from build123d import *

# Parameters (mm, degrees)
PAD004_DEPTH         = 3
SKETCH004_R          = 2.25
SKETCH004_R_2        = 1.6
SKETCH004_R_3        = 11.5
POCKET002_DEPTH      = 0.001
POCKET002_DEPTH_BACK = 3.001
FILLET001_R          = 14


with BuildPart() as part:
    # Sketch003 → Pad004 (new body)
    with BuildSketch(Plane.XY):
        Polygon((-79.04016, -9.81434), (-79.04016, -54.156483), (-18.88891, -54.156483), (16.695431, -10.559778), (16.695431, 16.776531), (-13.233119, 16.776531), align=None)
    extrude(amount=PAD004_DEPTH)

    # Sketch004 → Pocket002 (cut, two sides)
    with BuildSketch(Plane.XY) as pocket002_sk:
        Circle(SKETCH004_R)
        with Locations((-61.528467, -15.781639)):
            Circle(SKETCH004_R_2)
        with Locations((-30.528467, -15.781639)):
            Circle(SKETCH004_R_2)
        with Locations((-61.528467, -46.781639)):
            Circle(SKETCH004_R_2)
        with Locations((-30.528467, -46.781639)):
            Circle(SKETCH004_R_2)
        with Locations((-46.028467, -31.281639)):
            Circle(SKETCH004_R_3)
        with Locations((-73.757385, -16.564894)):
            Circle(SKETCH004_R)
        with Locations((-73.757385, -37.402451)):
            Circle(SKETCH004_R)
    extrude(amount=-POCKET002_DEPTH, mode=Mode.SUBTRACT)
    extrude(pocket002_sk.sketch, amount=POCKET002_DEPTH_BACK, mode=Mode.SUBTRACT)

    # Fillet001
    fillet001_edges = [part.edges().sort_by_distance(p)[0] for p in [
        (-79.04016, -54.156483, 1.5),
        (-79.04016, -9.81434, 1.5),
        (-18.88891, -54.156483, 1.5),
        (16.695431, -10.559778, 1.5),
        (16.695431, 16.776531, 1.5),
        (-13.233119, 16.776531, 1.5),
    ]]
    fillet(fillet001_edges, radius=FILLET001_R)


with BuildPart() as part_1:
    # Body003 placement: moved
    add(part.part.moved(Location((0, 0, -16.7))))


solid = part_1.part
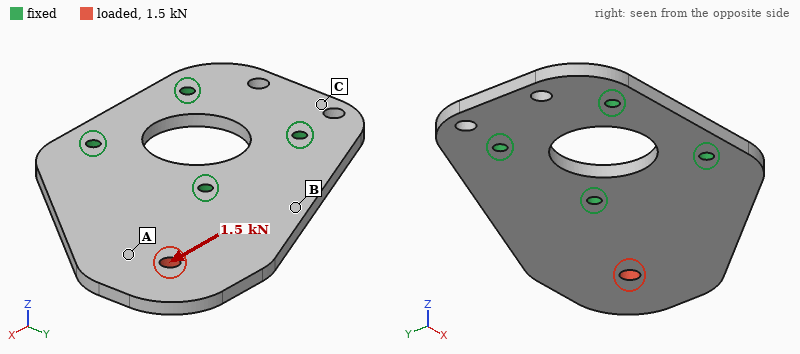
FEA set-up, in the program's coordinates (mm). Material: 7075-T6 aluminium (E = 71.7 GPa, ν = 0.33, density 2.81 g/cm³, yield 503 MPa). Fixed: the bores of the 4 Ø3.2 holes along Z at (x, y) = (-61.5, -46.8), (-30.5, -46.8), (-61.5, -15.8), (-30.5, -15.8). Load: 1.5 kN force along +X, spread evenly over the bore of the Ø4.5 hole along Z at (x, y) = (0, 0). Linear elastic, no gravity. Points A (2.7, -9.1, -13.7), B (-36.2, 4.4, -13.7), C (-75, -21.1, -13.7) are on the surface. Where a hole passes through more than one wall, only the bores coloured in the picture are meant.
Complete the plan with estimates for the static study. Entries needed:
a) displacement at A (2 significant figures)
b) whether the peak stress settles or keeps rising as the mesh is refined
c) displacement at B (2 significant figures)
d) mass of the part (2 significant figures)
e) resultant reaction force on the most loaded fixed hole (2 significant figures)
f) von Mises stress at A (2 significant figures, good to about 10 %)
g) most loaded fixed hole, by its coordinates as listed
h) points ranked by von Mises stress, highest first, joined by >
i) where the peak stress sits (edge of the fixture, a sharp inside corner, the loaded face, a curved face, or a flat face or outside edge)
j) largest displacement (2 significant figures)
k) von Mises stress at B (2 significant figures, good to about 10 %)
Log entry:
17 µm
keeps rising
9.6 µm
38 g
1.2 kN
11 MPa
(-30.5, -15.8)
B > A > C
edge of the fixture
26 µm
20 MPa
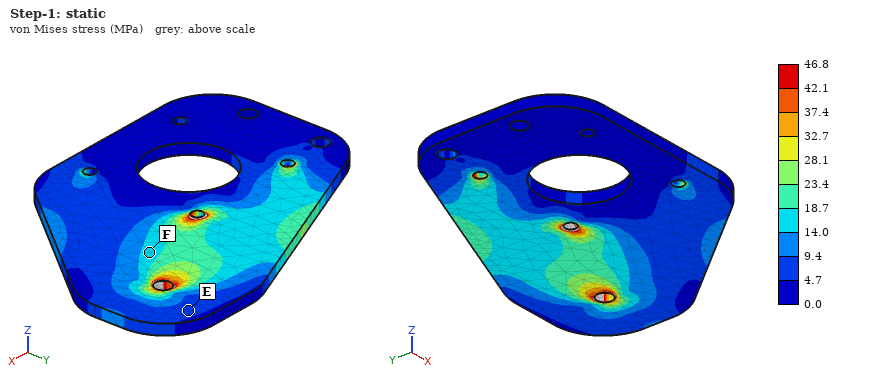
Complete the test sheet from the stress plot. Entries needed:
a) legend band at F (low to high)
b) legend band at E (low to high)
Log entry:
14.0 to 18.7 MPa
4.7 to 9.4 MPa
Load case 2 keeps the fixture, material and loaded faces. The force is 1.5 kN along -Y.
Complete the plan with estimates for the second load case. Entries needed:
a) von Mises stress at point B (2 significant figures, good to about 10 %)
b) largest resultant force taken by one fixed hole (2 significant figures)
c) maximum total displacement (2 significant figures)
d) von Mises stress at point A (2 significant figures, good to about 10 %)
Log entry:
20 MPa
1.2 kN
38 µm
23 MPa
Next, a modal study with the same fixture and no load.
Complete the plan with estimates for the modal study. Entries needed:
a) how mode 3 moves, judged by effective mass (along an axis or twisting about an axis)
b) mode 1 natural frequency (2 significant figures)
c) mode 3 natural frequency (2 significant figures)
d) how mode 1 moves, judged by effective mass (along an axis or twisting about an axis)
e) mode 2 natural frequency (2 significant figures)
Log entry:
along Z
1100 Hz
4600 Hz
along Z
2600 Hz
